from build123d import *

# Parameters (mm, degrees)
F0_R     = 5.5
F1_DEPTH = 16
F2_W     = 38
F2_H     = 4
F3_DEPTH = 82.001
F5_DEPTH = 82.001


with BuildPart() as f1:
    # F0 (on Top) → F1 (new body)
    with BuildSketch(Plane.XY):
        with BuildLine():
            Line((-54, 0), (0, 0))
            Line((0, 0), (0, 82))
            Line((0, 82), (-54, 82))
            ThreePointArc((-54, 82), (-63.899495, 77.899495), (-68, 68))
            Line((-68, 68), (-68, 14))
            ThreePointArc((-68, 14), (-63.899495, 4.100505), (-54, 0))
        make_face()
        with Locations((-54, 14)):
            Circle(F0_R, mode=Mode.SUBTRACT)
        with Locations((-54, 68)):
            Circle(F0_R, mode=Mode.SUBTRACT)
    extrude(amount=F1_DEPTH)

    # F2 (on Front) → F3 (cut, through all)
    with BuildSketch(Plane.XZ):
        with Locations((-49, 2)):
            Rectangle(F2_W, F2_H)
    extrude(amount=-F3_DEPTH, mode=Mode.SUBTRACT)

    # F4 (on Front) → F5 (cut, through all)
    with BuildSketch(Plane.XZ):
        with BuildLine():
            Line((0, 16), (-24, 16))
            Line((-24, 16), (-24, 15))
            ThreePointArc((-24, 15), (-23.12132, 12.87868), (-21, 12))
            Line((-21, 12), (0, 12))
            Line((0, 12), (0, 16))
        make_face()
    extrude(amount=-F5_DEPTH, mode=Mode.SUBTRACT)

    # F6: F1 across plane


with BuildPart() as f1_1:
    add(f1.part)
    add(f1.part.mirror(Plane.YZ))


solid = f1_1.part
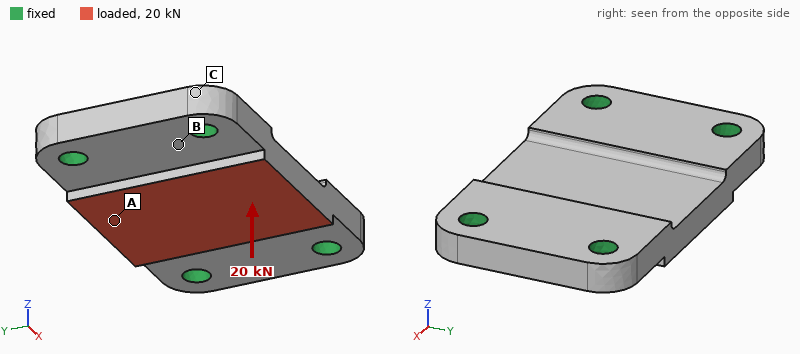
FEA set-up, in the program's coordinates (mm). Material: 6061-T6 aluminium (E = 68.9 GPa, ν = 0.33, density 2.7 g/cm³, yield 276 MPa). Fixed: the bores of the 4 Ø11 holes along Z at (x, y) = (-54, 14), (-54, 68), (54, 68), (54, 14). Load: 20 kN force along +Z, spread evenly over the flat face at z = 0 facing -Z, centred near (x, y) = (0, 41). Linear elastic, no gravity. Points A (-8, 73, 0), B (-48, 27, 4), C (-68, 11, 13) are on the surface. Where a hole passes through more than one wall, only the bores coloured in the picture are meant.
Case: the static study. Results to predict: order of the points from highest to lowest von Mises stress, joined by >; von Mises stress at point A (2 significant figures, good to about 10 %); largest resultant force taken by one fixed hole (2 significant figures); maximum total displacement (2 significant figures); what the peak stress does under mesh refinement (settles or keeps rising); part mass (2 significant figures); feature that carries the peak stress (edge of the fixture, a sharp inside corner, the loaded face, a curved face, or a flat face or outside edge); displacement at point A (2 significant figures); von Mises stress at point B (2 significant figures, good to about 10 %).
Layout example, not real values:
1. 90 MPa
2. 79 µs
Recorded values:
1. A > B > C
2. 66 MPa
3. 8.0 kN
4. 0.12 mm
5. keeps rising
6. 360 g
7. edge of the fixture
8. 0.11 mm
9. 34 MPa
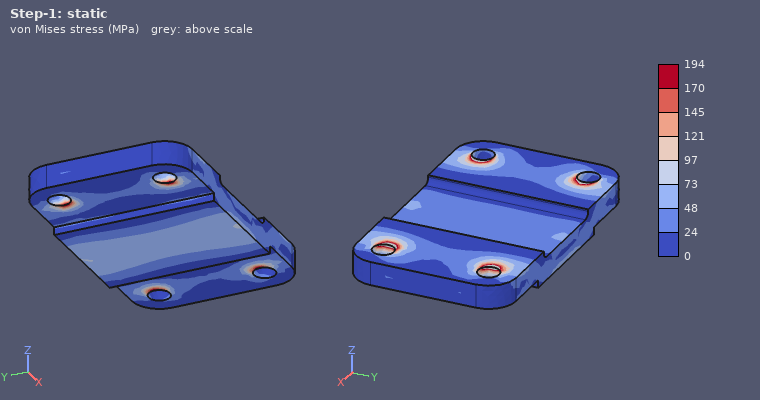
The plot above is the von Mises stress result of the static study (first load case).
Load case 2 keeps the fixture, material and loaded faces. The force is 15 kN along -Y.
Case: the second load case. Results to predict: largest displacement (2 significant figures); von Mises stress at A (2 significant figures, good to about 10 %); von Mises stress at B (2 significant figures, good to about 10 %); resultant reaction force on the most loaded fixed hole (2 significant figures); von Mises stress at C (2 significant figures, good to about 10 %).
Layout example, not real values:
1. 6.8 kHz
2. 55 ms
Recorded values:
1. 43 µm
2. 13 MPa
3. 21 MPa
4. 5.3 kN
5. 5.7 MPa
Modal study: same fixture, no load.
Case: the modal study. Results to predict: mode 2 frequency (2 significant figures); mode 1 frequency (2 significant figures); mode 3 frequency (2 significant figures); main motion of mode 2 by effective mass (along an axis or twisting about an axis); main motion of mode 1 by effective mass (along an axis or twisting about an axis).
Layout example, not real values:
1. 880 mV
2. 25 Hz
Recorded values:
1. 7000 Hz
2. 5400 Hz
3. 12 kHz
4. twisting about X
5. along Z
